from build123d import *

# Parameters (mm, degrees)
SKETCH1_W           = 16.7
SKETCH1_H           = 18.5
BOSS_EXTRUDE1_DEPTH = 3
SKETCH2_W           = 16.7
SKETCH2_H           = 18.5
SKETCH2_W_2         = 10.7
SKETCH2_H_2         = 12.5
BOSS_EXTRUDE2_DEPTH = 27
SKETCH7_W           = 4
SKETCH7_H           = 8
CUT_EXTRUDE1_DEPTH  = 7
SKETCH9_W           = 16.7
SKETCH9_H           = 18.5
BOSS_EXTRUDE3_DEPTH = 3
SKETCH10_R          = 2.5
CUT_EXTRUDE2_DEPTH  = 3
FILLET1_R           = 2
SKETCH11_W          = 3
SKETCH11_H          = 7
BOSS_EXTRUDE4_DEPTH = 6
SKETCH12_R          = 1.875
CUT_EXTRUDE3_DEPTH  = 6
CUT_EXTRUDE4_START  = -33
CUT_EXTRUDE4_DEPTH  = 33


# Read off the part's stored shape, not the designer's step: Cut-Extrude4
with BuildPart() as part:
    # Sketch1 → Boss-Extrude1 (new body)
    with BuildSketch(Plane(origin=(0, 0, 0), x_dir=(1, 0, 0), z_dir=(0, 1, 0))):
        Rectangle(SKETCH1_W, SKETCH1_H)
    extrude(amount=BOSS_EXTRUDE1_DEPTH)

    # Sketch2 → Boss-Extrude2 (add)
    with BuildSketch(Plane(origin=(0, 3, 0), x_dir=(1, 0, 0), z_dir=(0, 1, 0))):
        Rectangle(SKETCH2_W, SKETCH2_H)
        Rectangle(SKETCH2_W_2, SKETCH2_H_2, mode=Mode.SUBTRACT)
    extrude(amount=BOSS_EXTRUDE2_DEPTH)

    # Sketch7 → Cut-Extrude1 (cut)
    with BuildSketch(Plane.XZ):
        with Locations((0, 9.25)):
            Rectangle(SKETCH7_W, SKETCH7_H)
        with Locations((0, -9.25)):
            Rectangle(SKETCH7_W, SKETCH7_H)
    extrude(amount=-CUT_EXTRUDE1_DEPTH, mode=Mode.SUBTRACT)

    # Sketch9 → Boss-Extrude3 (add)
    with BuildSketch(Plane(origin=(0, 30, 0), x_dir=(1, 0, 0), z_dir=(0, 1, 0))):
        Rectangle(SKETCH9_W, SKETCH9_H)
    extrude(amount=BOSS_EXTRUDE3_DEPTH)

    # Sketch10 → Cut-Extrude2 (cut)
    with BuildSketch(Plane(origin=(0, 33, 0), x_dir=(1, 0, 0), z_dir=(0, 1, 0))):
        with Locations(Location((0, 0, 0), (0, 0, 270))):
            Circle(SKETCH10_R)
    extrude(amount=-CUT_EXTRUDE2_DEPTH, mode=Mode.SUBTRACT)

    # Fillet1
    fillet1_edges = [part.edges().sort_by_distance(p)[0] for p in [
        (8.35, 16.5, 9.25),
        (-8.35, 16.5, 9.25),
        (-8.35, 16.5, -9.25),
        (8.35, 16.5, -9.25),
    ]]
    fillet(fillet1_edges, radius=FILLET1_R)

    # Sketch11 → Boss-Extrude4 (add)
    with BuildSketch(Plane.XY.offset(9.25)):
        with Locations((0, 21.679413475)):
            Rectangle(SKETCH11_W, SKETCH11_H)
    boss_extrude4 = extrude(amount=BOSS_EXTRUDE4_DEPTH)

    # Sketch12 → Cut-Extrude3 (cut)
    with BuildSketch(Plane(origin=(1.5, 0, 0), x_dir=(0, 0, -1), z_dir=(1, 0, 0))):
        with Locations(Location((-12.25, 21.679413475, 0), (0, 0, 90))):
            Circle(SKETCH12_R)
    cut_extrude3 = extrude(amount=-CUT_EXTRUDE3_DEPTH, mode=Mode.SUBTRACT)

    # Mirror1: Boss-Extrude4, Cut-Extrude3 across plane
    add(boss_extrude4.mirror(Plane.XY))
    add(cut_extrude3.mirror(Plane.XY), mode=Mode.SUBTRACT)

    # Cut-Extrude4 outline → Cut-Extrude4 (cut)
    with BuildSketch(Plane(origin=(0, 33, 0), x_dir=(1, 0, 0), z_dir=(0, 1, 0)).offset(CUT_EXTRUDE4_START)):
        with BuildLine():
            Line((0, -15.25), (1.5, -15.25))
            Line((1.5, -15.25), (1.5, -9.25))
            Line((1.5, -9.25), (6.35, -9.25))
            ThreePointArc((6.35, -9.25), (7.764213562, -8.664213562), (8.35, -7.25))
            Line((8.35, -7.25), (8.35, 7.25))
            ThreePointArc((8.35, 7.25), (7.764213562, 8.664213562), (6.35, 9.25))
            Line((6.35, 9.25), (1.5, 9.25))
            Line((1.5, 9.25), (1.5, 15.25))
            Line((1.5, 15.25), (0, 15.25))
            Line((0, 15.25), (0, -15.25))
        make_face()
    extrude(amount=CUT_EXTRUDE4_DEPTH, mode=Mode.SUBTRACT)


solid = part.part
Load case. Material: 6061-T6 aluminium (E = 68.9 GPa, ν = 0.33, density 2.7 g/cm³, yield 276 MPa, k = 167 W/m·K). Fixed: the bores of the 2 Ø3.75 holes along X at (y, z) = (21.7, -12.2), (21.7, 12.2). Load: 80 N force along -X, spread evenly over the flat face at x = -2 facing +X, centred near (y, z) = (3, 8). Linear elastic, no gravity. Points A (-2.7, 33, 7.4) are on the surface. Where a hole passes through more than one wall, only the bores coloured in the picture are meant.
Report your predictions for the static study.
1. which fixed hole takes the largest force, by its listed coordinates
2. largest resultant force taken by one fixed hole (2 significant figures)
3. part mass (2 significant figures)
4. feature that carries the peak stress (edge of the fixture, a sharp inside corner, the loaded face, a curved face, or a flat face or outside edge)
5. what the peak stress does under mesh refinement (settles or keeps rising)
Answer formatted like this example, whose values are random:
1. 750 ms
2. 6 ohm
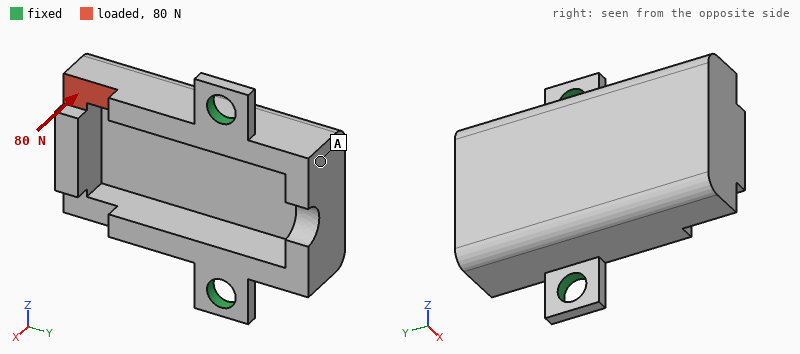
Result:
1. (21.7, 12.2)
2. 75 N
3. 8.6 g
4. edge of the fixture
5. keeps rising
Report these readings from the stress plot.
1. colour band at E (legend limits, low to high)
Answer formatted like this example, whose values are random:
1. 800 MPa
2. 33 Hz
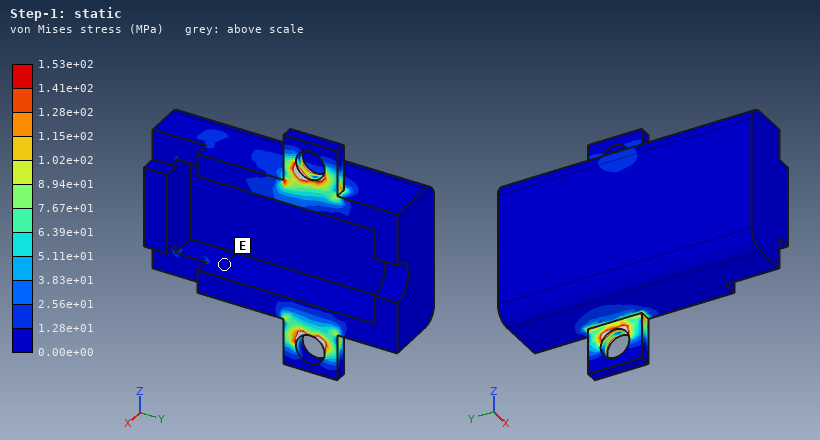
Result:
1. 0.00e+00 to 1.28e+01 MPa
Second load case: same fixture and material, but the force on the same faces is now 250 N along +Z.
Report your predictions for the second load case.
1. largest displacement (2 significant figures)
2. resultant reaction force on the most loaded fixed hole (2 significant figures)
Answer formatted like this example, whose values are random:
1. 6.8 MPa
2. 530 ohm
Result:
1. 49 µm
2. 230 N
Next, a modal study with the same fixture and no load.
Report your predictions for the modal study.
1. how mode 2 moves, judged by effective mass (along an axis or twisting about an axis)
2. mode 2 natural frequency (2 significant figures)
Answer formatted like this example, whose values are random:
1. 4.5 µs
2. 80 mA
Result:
1. along Z
2. 8900 Hz
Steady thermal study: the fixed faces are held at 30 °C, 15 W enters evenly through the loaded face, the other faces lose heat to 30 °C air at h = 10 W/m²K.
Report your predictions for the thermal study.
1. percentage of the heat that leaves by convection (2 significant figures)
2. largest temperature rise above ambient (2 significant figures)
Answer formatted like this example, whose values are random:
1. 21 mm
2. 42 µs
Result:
1. 3.2 %
2. 48 K
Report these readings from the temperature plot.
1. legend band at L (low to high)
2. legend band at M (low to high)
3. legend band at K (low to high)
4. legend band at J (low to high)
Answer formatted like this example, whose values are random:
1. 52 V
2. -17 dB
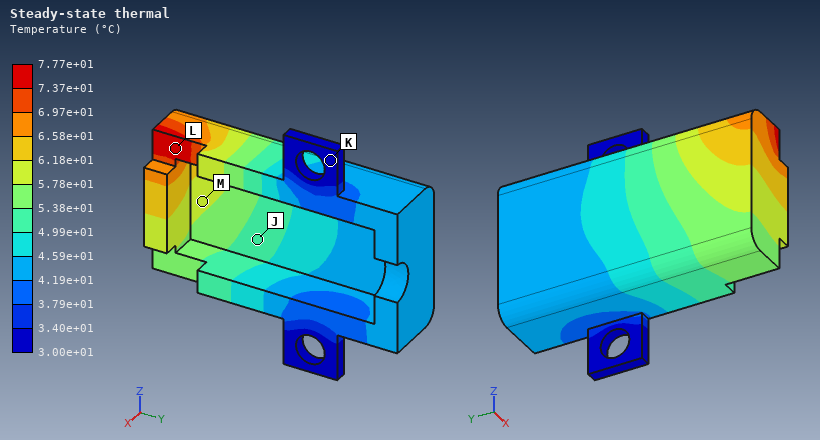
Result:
1. 7.37e+01 to 7.77e+01 °C
2. 5.78e+01 to 6.18e+01 °C
3. 3.00e+01 to 3.40e+01 °C
4. 4.99e+01 to 5.38e+01 °C
